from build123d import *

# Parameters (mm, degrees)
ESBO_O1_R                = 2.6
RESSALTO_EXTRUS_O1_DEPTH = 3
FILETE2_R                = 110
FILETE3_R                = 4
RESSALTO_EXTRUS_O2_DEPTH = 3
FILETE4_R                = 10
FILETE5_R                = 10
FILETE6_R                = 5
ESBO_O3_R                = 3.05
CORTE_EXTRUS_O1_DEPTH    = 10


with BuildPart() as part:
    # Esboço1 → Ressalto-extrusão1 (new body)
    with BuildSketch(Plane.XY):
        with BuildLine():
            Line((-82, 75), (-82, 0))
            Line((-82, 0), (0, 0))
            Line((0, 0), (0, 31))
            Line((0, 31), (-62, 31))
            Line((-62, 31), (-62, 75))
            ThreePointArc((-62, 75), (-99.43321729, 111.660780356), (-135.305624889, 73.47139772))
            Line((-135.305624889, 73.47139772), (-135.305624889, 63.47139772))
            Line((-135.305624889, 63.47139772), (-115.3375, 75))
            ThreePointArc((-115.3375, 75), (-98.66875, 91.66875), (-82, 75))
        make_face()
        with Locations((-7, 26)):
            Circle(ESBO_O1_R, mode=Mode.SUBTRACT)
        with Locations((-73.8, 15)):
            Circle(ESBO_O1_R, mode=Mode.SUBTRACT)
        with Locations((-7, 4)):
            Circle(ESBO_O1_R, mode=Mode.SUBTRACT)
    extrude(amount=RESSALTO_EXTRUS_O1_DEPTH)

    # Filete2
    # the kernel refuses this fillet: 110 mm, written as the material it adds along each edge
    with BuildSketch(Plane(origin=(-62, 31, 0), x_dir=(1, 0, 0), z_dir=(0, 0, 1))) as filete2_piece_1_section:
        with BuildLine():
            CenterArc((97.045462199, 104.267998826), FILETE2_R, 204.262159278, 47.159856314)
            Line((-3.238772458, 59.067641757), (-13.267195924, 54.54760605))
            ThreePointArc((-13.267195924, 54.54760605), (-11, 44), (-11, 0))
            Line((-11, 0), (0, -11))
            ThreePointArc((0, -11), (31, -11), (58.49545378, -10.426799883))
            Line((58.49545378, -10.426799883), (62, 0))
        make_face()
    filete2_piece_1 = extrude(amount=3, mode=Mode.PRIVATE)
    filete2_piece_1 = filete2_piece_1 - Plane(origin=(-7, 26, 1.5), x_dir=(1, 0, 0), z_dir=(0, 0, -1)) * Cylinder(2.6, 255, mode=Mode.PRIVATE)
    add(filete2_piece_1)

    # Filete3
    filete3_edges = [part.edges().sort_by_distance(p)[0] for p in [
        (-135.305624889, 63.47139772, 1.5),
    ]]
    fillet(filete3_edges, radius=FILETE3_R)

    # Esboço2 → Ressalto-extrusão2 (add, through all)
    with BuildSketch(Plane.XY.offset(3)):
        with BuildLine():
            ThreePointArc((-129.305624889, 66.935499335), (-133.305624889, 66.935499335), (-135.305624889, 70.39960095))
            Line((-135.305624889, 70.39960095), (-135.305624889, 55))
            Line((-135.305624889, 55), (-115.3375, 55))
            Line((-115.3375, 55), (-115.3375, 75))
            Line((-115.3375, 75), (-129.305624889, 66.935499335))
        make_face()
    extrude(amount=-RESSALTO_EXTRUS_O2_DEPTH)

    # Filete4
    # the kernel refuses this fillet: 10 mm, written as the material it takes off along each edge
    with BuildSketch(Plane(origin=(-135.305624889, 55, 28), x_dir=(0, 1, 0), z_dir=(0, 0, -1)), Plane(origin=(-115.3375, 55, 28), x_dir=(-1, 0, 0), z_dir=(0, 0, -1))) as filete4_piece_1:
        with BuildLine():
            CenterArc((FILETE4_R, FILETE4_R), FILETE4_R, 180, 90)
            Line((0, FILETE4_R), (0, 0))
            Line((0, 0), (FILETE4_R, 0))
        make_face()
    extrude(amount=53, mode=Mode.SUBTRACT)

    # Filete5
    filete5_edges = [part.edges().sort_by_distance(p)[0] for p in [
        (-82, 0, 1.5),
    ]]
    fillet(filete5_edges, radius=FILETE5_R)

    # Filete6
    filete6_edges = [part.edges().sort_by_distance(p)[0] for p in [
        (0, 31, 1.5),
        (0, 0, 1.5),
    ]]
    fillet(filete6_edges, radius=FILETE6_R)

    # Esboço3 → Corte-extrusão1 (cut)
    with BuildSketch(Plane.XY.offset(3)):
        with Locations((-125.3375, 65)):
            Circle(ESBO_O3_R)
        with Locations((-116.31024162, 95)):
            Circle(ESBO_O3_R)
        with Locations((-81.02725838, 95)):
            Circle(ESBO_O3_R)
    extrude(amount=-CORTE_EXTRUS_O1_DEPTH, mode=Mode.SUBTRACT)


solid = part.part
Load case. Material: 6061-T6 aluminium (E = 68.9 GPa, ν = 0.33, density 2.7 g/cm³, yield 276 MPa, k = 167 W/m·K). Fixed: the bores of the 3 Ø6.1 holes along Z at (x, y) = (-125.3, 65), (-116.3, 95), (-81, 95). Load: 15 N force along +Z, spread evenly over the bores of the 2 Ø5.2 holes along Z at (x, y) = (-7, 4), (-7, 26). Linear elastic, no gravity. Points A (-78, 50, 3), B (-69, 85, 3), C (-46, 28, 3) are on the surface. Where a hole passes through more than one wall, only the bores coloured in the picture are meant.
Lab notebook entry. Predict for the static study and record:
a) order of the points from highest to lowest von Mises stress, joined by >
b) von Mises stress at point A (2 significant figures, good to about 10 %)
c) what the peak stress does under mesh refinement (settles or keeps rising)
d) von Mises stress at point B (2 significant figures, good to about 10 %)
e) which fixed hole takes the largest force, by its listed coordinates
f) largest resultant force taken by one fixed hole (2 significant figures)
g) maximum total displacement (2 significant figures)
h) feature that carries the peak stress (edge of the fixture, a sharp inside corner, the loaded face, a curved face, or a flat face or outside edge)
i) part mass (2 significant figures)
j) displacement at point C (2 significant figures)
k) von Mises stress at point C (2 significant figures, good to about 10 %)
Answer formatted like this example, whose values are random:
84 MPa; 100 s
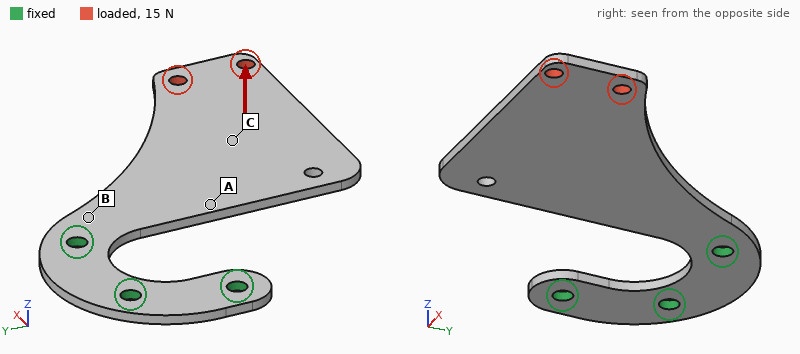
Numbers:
B > A > C; 17 MPa; keeps rising; 42 MPa; (-81, 95); 18 N; 1.8 mm; edge of the fixture; 53 g; 0.85 mm; 7.4 MPa
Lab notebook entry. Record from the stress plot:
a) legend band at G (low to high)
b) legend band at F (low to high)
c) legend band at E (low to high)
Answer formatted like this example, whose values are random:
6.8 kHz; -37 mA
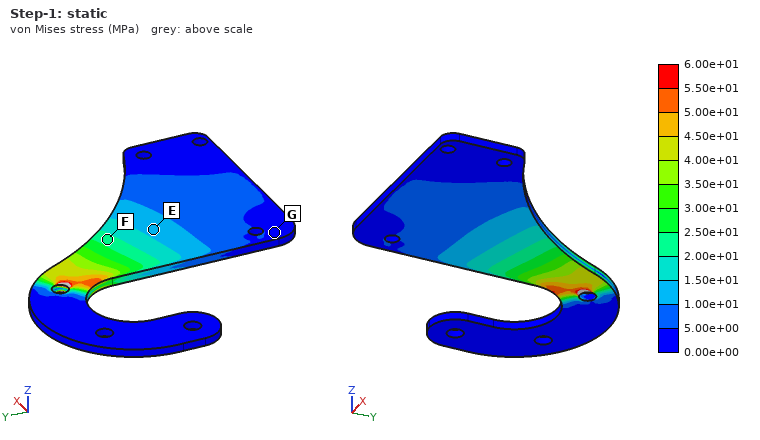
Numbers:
0.00e+00 to 5.00e+00 MPa; 2.00e+01 to 2.50e+01 MPa; 1.00e+01 to 1.50e+01 MPa
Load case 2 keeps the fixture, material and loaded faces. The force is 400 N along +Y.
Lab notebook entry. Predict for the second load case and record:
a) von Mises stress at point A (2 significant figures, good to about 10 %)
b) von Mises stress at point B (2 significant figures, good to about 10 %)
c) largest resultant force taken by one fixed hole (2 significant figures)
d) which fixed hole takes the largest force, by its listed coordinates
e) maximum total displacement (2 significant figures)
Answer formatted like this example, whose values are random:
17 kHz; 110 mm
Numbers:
21 MPa; 69 MPa; 880 N; (-81, 95); 0.83 mm
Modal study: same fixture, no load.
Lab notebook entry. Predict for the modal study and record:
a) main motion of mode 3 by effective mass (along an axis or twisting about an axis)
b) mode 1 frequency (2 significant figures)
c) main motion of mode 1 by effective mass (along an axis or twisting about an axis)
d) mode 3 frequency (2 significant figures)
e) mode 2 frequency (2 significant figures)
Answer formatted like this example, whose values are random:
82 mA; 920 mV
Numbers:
along X; 130 Hz; along Z; 760 Hz; 450 Hz
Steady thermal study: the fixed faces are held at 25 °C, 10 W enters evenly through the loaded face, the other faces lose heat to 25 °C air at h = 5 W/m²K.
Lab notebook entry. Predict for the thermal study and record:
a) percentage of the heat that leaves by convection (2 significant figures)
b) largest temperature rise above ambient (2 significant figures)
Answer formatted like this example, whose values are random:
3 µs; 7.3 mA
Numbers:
20 %; 63 K
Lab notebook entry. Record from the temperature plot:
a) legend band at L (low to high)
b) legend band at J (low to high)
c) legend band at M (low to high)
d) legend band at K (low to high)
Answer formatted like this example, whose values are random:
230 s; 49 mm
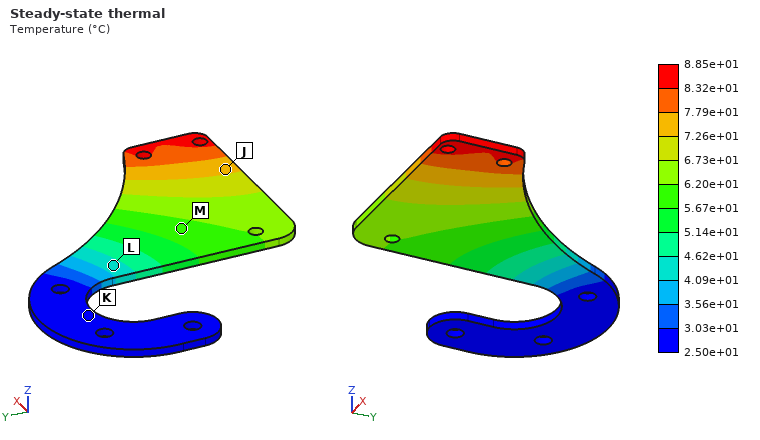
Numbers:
4.09e+01 to 4.62e+01 °C; 7.26e+01 to 7.79e+01 °C; 5.67e+01 to 6.20e+01 °C; 2.50e+01 to 3.03e+01 °C
